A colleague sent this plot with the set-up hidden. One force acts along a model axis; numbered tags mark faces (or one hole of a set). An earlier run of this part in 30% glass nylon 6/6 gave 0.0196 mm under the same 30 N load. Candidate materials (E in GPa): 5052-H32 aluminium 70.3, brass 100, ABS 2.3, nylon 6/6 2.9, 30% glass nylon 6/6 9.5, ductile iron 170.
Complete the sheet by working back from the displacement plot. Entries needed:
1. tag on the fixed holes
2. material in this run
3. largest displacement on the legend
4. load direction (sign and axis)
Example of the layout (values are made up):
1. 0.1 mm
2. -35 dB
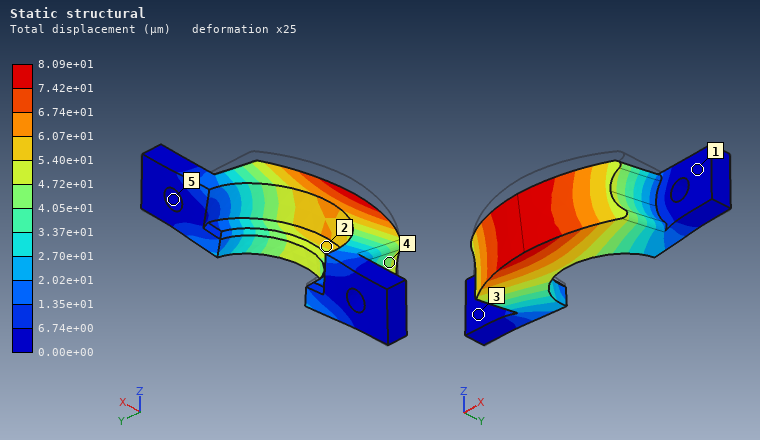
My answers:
1. 5
2. ABS
3. 8.09e+01 µm
4. -Z
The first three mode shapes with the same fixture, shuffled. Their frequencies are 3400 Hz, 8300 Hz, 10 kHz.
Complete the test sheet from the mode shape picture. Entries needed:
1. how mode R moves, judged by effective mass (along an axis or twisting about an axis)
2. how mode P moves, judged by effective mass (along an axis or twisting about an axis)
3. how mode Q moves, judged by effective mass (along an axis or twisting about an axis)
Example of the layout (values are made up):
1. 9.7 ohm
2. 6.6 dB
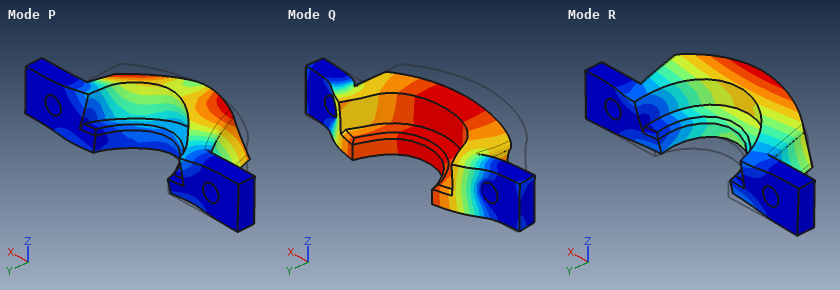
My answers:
1. along Z
2. along X
3. along Y
